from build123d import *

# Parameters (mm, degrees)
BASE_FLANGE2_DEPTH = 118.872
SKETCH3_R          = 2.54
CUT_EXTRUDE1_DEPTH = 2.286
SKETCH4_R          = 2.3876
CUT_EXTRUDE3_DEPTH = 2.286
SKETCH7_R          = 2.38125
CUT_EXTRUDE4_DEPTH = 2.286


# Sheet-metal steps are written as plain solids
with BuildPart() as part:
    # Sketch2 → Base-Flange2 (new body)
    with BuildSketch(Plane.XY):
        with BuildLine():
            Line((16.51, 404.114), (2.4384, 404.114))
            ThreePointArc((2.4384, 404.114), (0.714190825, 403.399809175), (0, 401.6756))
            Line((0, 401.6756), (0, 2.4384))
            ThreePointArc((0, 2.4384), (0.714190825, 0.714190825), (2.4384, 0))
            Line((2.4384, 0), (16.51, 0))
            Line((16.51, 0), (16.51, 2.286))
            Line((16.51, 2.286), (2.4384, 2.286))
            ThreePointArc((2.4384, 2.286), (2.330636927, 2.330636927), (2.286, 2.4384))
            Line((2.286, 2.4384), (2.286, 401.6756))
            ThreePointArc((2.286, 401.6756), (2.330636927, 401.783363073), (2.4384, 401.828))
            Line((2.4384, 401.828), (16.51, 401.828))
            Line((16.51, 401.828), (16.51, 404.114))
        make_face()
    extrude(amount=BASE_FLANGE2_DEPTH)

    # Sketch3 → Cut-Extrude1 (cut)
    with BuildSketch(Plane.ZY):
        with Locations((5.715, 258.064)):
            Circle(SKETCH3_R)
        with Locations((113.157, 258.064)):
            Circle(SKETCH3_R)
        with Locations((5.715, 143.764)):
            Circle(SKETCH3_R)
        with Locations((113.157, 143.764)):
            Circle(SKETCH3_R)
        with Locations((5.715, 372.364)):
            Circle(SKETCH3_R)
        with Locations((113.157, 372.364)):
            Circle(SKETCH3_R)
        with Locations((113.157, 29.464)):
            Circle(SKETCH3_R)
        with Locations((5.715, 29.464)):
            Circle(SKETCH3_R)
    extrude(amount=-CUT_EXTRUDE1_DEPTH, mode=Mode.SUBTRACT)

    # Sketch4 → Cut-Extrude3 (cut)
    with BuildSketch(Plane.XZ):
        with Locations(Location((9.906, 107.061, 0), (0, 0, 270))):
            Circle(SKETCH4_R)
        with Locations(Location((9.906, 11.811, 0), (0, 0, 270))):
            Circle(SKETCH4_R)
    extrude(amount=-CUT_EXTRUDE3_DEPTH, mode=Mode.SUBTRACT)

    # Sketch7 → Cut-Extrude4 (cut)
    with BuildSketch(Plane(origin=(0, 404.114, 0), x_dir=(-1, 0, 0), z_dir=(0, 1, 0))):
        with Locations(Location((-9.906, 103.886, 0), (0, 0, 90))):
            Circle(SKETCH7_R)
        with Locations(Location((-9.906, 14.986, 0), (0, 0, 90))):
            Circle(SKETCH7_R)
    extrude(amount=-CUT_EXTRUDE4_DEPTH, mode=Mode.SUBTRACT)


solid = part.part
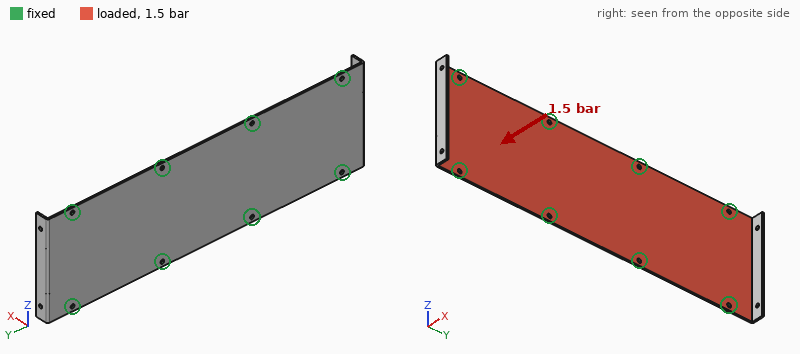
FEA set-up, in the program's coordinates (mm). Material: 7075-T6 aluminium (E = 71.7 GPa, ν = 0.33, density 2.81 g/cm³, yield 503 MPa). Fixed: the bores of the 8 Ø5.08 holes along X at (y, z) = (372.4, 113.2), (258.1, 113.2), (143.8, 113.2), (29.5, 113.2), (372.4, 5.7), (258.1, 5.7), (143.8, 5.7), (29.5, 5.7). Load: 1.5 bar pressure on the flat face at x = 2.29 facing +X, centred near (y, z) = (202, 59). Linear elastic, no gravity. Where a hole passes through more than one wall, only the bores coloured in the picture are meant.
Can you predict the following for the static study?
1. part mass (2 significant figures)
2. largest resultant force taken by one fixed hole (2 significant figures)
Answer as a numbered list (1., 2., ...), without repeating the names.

1. 330 g
2. 1.0 kN
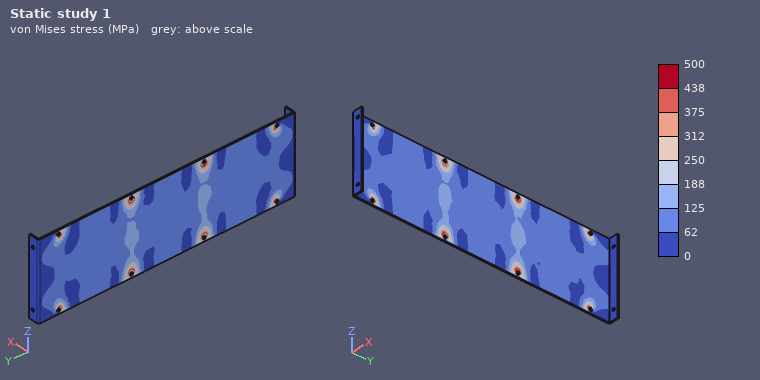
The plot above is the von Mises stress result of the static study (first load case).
